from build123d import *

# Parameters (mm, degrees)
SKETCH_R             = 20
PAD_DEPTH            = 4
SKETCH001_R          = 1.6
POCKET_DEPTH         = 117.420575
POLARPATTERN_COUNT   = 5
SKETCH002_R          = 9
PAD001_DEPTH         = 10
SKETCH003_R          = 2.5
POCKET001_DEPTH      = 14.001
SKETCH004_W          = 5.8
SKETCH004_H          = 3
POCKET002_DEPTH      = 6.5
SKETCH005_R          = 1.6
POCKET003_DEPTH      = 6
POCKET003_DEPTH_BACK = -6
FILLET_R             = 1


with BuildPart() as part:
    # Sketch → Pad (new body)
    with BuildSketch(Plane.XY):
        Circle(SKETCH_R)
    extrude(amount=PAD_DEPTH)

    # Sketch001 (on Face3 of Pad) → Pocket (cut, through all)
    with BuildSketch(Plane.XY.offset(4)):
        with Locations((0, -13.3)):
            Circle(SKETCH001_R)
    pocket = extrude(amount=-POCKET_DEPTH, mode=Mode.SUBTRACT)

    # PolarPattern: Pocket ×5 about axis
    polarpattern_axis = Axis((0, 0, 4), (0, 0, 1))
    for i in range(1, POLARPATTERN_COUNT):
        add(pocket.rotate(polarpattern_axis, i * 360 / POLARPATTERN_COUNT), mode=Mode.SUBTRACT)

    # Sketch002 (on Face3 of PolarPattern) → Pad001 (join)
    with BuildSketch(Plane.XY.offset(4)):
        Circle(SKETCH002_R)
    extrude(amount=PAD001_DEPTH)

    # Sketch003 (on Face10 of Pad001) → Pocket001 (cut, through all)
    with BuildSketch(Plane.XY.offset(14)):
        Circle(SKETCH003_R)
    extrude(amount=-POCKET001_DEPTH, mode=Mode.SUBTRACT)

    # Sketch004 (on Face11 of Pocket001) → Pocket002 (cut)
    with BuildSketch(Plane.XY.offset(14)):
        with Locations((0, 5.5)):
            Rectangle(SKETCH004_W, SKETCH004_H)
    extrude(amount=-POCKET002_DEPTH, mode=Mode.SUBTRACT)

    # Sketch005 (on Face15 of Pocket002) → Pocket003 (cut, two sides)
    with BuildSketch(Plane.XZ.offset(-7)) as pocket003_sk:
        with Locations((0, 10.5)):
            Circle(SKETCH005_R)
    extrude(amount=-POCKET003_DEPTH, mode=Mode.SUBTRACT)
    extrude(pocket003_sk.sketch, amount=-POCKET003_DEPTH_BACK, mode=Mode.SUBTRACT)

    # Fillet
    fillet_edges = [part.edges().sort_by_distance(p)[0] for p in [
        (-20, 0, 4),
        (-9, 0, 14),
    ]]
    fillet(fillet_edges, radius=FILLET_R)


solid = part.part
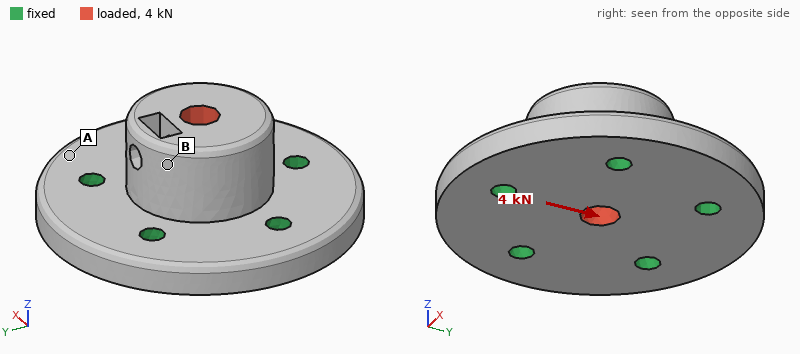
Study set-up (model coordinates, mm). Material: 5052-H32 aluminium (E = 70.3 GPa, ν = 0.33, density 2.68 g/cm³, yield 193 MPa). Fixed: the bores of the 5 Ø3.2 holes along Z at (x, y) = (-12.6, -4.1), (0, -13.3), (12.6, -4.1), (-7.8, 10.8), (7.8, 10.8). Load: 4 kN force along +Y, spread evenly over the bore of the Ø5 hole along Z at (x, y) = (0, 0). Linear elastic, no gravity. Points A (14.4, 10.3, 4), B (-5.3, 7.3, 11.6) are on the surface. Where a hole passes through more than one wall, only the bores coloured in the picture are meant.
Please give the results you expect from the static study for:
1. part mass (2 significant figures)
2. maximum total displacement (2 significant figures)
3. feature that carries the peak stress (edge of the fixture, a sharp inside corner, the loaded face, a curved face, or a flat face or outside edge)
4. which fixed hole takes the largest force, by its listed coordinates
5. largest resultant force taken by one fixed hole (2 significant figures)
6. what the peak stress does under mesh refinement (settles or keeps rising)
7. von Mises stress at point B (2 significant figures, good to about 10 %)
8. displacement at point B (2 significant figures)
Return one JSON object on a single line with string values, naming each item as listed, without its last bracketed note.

{"part mass": "19 g", "maximum total displacement": "15 µm", "feature that carries the peak stress": "edge of the fixture", "which fixed hole takes the largest force, by its listed coordinates": "(0, -13.3)", "largest resultant force taken by one fixed hole": "1.3 kN", "what the peak stress does under mesh refinement": "keeps rising", "von Mises stress at point B": "15 MPa", "displacement at point B": "11 µm"}
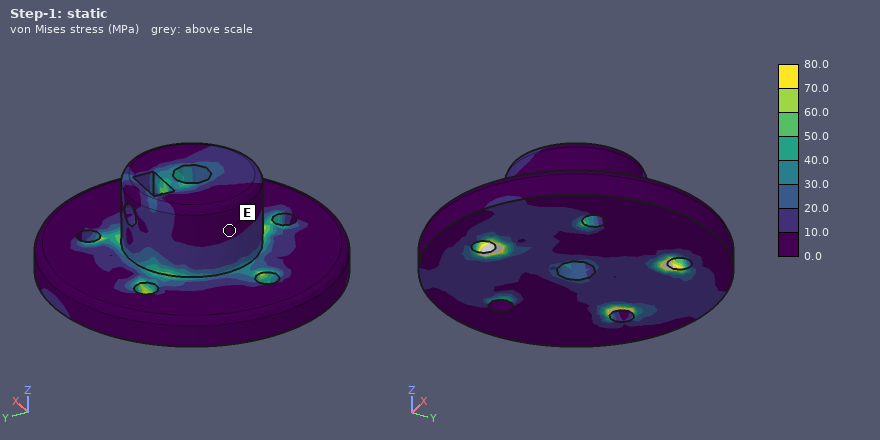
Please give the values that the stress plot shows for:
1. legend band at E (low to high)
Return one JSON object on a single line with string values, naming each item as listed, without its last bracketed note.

{"legend band at E": "0.0 to 10.0 MPa"}
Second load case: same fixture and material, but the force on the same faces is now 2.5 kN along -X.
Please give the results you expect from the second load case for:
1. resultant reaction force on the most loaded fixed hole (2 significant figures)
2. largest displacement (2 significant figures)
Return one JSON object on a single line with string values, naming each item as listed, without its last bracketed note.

{"resultant reaction force on the most loaded fixed hole": "800 N", "largest displacement": "8.6 µm"}
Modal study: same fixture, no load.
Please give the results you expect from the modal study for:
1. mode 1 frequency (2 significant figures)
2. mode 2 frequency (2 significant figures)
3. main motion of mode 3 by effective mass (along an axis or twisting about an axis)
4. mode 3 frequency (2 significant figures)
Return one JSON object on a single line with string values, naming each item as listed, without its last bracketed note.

{"mode 1 frequency": "34 kHz", "mode 2 frequency": "34 kHz", "main motion of mode 3 by effective mass": "along Z", "mode 3 frequency": "37 kHz"}
